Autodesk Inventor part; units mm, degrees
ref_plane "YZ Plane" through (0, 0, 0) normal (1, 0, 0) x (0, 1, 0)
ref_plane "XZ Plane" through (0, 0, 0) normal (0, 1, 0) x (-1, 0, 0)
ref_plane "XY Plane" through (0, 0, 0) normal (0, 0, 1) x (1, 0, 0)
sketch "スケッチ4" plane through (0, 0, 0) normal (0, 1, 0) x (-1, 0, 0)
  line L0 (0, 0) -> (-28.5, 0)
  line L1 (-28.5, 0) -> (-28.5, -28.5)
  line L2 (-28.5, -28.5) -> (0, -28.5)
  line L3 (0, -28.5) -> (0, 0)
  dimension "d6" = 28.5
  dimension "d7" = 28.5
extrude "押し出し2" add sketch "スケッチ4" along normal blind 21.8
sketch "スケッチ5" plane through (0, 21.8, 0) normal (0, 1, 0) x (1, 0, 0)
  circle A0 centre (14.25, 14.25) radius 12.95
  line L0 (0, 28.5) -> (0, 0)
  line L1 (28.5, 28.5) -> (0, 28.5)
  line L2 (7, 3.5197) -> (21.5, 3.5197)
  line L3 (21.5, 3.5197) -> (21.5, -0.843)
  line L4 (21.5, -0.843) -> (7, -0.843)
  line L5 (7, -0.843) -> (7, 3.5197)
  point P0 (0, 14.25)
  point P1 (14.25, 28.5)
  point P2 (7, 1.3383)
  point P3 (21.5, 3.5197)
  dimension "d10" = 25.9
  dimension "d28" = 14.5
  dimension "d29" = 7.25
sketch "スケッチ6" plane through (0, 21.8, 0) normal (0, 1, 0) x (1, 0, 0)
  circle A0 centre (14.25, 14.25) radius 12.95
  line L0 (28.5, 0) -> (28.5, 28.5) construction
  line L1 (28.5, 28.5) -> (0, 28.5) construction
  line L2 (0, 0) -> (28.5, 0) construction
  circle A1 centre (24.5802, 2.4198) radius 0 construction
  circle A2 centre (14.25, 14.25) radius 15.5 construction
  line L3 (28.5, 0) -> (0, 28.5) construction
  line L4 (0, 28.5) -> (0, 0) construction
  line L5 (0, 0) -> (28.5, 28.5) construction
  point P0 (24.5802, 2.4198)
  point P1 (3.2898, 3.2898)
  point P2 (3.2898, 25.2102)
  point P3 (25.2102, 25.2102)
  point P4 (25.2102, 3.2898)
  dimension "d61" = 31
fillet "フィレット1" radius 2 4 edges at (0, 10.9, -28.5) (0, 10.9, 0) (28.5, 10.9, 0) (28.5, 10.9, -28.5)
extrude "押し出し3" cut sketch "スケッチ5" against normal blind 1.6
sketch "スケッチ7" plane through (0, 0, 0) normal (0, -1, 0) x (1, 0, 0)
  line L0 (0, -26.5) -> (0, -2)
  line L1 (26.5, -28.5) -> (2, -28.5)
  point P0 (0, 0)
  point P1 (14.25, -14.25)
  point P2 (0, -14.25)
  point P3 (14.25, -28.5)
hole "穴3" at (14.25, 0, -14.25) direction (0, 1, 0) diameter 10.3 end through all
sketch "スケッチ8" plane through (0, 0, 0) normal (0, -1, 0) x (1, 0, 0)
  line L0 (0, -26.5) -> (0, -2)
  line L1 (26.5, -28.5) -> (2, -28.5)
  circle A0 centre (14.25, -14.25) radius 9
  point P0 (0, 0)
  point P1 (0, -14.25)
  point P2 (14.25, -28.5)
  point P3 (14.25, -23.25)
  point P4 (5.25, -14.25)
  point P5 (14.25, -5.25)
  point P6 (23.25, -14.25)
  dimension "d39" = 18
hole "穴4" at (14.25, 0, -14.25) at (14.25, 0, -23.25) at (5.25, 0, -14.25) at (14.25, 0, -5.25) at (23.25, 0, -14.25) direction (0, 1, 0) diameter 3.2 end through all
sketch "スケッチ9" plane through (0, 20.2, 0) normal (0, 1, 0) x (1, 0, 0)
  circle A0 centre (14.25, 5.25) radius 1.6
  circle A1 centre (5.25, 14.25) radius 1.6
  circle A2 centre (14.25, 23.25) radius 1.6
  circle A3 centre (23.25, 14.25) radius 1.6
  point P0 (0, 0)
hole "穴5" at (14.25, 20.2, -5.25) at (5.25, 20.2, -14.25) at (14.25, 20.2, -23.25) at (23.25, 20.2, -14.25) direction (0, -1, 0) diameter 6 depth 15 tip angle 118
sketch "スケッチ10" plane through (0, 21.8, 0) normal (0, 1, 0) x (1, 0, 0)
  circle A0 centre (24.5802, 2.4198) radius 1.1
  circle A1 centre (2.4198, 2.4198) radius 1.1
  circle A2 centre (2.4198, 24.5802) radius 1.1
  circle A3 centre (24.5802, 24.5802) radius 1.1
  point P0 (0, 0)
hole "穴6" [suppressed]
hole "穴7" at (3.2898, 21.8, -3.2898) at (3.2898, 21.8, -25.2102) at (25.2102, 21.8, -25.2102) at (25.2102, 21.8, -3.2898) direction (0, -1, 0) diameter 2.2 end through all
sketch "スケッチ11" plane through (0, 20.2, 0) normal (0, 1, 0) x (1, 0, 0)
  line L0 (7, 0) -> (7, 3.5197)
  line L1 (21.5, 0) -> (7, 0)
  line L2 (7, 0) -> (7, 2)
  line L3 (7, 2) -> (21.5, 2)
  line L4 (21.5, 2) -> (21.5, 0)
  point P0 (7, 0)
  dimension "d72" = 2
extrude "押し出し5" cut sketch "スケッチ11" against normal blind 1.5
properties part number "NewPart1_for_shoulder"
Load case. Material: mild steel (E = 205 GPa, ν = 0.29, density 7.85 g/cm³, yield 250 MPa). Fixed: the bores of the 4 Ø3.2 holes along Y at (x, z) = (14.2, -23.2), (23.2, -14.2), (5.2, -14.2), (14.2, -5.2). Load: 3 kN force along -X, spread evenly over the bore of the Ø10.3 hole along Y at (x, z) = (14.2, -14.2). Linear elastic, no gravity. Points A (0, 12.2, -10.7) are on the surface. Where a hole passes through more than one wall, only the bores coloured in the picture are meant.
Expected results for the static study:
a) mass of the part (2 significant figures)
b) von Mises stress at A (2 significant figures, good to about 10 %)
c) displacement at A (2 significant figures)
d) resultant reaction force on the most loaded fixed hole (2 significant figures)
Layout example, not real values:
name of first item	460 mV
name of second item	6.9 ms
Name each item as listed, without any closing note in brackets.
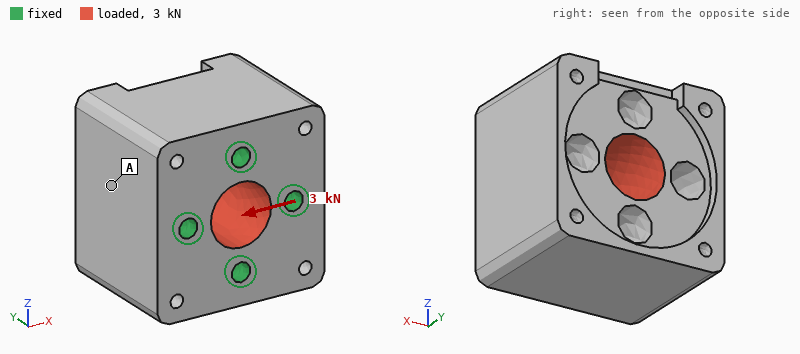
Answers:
mass of the part	100 g
von Mises stress at A	8.7 MPa
displacement at A	2.4 µm
resultant reaction force on the most loaded fixed hole	1.2 kN
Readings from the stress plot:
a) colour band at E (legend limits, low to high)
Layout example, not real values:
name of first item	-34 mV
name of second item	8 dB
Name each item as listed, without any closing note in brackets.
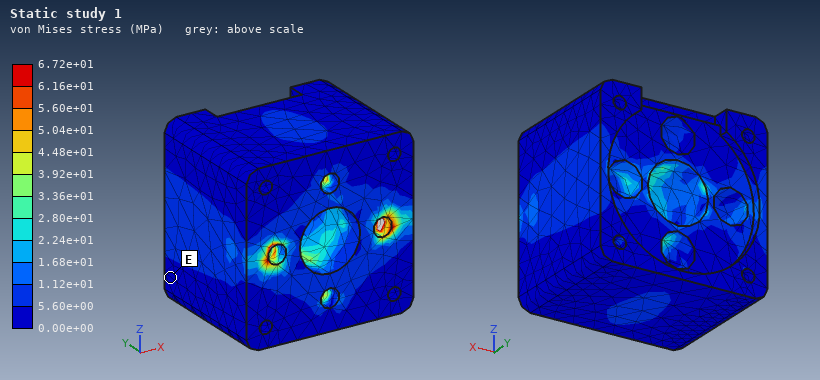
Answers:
colour band at E	0.00e+00 to 5.60e+00 MPa
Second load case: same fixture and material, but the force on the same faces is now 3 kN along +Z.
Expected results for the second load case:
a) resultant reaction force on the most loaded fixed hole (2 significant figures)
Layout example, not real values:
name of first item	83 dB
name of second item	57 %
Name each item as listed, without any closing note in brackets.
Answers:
resultant reaction force on the most loaded fixed hole	1.2 kN
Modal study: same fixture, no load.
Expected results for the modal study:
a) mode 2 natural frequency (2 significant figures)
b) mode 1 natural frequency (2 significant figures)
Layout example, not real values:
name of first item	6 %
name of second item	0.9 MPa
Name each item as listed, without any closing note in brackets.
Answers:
mode 2 natural frequency	16 kHz
mode 1 natural frequency	16 kHz
